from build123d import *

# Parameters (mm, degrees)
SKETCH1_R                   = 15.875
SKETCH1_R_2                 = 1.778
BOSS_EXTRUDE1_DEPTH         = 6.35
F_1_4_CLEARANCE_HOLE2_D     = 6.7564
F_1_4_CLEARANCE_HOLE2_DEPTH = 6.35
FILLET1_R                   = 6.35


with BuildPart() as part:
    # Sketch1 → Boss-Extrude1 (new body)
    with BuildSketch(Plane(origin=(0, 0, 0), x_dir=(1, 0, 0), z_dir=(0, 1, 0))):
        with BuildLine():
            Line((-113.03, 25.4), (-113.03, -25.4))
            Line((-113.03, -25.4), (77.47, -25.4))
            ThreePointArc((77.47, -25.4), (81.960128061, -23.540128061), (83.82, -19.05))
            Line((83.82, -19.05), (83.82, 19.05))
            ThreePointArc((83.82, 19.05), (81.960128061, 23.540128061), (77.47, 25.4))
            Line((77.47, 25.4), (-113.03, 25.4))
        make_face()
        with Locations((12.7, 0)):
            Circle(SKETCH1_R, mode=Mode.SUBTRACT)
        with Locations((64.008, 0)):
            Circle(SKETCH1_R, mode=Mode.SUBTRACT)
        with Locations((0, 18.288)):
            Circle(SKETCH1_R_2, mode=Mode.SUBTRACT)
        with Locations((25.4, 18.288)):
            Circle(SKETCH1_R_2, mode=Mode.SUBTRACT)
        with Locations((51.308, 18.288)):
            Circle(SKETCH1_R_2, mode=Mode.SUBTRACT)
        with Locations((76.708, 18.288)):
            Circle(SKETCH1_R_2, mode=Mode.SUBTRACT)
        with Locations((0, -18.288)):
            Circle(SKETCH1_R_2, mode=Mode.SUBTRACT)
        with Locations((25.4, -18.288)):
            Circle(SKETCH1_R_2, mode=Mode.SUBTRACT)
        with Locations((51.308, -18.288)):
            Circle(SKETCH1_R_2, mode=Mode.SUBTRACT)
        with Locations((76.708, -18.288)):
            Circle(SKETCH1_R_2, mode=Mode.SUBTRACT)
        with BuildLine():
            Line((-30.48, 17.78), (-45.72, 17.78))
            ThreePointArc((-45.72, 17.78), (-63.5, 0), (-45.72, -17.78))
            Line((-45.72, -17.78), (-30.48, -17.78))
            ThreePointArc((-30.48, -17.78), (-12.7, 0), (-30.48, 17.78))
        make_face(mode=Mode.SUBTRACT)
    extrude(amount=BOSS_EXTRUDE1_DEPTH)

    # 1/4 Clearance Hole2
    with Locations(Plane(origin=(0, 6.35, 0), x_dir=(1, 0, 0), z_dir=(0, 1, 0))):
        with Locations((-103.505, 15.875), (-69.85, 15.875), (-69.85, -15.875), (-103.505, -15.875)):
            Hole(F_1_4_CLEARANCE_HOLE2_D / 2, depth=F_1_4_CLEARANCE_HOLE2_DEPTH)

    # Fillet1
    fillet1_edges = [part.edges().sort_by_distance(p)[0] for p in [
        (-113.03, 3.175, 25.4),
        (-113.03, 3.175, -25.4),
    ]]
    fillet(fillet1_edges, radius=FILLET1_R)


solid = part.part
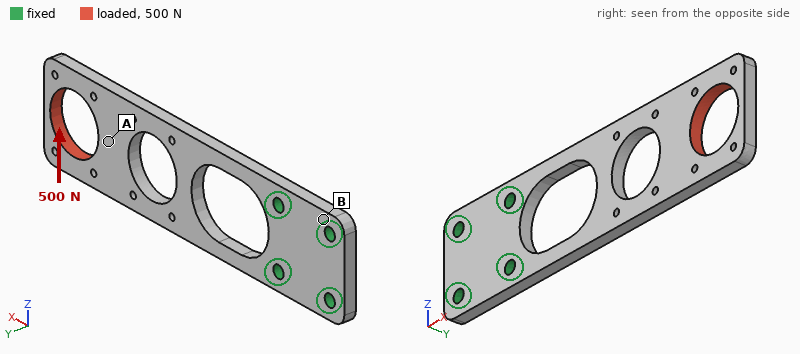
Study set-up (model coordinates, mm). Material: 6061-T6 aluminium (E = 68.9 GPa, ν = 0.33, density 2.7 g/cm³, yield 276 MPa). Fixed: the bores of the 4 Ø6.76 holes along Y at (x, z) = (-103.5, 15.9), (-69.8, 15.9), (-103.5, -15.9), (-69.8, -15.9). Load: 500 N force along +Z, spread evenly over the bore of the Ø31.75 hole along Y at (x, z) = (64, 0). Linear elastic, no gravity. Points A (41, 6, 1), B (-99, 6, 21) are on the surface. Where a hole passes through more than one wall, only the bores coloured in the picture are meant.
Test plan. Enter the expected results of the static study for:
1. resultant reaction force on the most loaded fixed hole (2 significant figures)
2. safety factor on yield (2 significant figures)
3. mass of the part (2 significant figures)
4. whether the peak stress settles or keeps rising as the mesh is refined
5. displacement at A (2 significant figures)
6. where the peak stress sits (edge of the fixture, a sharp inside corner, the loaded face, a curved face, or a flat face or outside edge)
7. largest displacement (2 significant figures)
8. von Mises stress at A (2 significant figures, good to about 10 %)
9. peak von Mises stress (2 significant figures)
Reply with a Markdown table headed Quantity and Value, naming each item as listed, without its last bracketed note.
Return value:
| Quantity | Value |
|---|---|
| resultant reaction force on the most loaded fixed hole | 1.4 kN |
| safety factor on yield | 3.9 |
| mass of the part | 110 g |
| whether the peak stress settles or keeps rising as the mesh is refined | settles |
| displacement at A | 0.21 mm |
| where the peak stress sits | a flat face or outside edge |
| largest displacement | 0.29 mm |
| von Mises stress at A | 11 MPa |
| peak von Mises stress | 70 MPa |
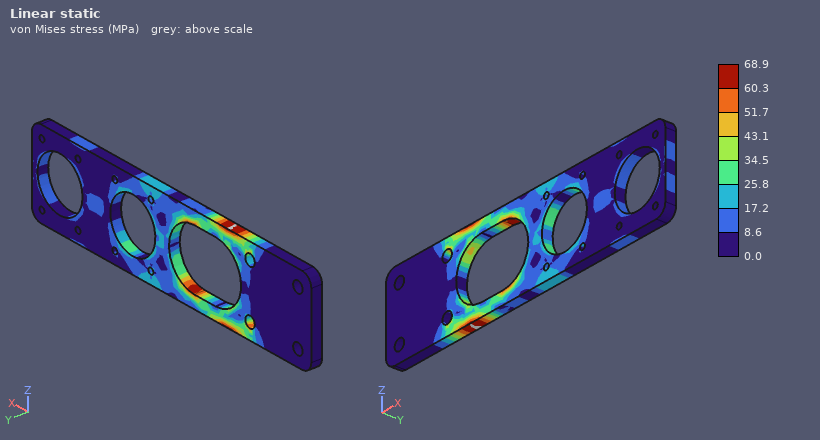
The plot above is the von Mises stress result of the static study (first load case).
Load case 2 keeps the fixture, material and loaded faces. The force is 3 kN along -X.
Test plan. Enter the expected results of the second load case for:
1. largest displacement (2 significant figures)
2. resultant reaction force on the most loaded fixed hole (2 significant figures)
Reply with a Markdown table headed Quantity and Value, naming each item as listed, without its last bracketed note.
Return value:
| Quantity | Value |
|---|---|
| largest displacement | 69 µm |
| resultant reaction force on the most loaded fixed hole | 1.4 kN |
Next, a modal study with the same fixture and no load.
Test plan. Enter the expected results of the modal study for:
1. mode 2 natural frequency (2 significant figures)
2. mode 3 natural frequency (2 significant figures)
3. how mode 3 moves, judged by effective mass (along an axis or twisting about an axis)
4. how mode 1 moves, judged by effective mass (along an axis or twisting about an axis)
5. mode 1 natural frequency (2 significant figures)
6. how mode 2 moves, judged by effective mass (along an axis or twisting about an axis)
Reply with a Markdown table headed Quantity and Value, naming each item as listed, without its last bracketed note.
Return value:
| Quantity | Value |
|---|---|
| mode 2 natural frequency | 930 Hz |
| mode 3 natural frequency | 1100 Hz |
| how mode 3 moves, judged by effective mass | along Z |
| how mode 1 moves, judged by effective mass | along Y |
| mode 1 natural frequency | 180 Hz |
| how mode 2 moves, judged by effective mass | twisting about X |
